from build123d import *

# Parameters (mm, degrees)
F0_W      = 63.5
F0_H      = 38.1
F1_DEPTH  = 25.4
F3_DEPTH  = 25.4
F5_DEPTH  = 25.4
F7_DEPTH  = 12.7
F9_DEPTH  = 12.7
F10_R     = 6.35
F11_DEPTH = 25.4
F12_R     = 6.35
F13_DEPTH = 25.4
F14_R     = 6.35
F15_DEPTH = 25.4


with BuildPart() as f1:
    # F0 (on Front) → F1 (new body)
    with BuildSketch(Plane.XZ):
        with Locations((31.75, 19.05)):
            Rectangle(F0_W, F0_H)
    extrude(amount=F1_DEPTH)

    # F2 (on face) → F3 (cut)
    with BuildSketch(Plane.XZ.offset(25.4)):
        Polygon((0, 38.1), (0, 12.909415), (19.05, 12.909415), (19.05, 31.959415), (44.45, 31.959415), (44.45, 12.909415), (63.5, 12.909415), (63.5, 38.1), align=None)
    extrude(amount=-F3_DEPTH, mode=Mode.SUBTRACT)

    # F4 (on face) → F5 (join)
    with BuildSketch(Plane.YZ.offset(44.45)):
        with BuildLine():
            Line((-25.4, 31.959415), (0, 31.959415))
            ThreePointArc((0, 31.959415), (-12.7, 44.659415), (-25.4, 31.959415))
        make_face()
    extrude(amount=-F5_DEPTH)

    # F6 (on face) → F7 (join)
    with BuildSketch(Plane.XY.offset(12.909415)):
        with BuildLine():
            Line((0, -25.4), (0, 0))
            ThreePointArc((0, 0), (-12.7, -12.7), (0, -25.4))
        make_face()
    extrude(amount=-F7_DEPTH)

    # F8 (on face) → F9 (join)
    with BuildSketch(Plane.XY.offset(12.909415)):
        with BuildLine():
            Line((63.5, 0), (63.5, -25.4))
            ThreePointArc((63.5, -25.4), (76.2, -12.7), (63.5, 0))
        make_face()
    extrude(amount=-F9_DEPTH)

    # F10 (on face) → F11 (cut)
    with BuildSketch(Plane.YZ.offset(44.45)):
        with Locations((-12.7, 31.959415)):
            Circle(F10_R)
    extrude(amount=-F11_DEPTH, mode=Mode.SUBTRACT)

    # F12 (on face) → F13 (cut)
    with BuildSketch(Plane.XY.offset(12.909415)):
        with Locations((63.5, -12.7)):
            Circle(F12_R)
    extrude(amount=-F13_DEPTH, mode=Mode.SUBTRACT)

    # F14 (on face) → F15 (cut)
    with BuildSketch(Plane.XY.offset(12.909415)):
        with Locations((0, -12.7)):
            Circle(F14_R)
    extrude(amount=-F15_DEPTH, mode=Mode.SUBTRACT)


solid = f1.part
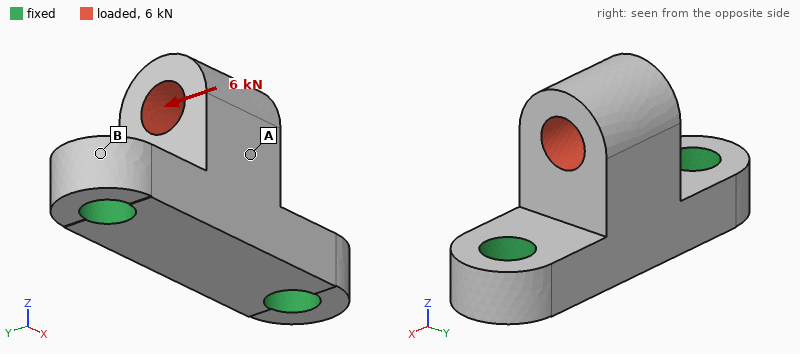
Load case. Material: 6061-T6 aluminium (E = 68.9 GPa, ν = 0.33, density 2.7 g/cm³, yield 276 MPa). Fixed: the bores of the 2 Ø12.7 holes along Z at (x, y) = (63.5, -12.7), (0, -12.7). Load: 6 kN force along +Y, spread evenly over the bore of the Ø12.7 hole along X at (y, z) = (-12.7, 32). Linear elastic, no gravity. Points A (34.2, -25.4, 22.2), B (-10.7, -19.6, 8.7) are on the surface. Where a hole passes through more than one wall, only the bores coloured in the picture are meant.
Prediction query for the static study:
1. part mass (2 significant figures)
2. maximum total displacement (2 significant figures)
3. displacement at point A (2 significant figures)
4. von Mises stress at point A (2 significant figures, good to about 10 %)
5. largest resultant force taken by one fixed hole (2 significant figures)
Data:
110 g
0.19 mm
0.096 mm
31 MPa
3.0 kN
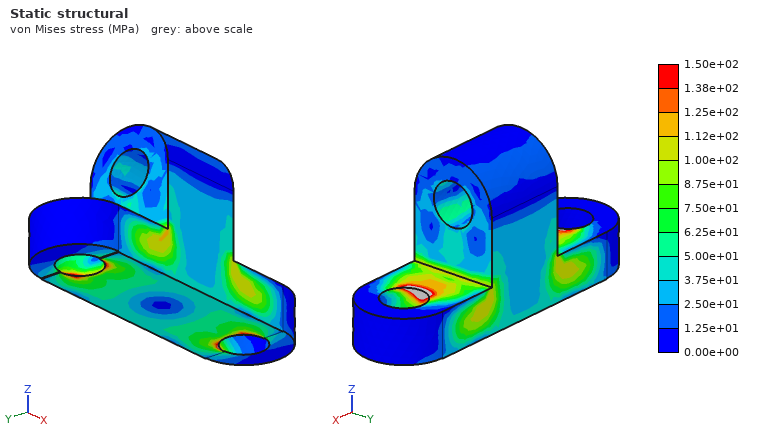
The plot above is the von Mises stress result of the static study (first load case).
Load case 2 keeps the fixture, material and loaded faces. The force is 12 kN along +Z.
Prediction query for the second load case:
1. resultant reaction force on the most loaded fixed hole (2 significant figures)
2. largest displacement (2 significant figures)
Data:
6.3 kN
41 µm
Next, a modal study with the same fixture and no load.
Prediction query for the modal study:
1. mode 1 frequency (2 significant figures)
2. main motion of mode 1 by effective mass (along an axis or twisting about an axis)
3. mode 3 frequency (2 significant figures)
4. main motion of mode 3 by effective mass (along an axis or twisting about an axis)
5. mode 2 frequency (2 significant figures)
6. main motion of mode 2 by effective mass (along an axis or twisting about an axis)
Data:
5700 Hz
along Y
12 kHz
along Z
11 kHz
along X
